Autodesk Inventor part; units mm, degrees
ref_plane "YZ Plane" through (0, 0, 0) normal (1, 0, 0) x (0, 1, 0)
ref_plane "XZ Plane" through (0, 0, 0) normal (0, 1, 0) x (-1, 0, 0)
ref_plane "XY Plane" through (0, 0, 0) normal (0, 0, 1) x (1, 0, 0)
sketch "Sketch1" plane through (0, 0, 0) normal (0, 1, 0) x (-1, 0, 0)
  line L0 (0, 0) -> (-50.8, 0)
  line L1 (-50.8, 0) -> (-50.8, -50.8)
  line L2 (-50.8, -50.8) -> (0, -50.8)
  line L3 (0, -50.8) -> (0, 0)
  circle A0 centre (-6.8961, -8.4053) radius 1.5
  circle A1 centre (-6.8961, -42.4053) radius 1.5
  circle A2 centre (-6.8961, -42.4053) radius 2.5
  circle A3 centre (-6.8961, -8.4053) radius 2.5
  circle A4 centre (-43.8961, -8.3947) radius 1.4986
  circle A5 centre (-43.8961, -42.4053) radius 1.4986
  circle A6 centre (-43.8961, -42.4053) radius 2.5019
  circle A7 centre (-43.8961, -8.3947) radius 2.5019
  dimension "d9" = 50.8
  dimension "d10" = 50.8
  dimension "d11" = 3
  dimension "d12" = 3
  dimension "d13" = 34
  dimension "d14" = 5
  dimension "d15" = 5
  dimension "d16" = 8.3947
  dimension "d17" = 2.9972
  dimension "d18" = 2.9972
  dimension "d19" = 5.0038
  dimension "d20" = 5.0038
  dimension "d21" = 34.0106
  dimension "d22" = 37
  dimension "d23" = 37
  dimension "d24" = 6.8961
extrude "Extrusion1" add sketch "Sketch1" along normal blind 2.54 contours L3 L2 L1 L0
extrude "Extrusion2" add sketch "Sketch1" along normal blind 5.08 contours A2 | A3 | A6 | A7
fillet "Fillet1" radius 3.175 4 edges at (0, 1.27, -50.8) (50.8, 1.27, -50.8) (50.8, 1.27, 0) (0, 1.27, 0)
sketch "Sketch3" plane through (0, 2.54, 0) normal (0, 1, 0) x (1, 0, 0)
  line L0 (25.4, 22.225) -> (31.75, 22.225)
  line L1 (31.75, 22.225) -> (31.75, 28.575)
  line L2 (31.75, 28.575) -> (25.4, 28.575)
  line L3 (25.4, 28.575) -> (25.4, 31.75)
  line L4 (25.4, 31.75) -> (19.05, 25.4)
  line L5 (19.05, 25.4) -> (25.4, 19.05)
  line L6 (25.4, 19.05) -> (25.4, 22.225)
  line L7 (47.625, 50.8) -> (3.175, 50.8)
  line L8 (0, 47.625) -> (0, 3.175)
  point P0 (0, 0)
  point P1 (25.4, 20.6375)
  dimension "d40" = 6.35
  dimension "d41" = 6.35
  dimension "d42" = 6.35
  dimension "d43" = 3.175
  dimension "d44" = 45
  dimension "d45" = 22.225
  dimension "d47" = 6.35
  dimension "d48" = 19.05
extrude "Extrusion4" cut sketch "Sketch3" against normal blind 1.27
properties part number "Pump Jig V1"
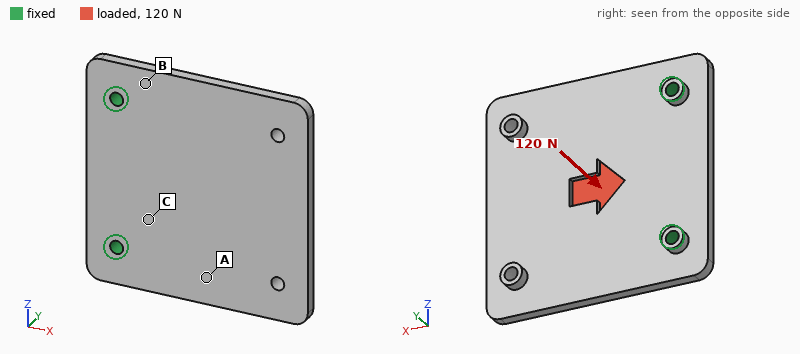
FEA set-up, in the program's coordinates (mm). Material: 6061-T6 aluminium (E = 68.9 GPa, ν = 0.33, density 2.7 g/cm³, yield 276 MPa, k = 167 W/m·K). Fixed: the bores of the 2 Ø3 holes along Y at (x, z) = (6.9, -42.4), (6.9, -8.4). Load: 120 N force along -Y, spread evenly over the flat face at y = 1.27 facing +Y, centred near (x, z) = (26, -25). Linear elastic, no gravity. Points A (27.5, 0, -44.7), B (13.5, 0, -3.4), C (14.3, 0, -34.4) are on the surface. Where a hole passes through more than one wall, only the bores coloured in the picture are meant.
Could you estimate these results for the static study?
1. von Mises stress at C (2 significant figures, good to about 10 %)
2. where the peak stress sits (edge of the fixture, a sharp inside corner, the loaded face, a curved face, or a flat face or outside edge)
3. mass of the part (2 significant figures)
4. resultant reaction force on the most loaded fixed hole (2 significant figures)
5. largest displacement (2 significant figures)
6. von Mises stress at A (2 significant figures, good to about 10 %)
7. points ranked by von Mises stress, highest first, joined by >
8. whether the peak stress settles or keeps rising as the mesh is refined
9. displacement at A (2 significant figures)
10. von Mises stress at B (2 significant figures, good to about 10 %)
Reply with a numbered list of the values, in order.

1. 22 MPa
2. edge of the fixture
3. 18 g
4. 62 N
5. 0.22 mm
6. 6.6 MPa
7. B > C > A
8. keeps rising
9. 0.071 mm
10. 33 MPa
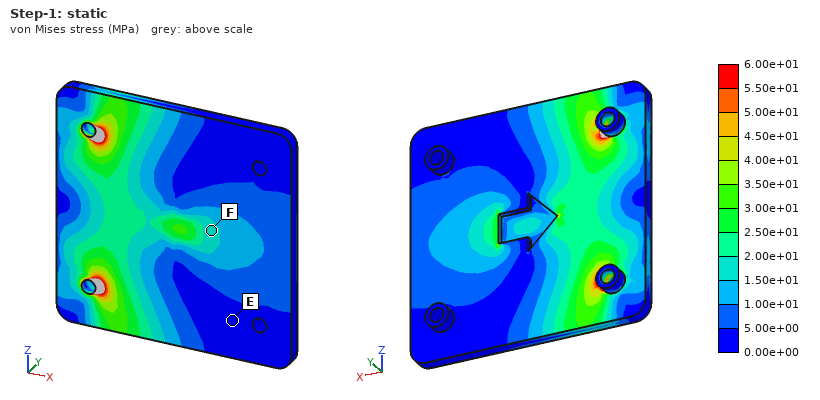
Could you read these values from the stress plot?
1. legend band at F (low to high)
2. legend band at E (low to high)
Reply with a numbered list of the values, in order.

1. 1.50e+01 to 2.00e+01 MPa
2. 0.00e+00 to 5.00e+00 MPa
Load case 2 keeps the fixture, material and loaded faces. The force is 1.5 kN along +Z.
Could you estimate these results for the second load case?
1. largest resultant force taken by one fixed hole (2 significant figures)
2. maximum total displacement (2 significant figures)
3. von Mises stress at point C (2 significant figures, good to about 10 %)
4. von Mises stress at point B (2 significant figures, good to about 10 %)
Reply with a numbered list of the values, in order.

1. 1.1 kN
2. 23 µm
3. 29 MPa
4. 13 MPa
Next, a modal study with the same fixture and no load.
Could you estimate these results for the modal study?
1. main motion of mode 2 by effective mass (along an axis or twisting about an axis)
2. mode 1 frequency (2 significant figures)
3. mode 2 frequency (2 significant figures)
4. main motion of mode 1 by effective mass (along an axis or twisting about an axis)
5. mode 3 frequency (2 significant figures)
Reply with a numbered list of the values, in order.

1. twisting about X
2. 1000 Hz
3. 2300 Hz
4. along Y
5. 6100 Hz
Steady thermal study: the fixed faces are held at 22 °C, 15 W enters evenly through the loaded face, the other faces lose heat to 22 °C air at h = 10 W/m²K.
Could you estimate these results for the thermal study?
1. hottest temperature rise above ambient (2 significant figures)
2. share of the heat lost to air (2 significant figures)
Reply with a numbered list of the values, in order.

1. 25 K
2. 4.6 %
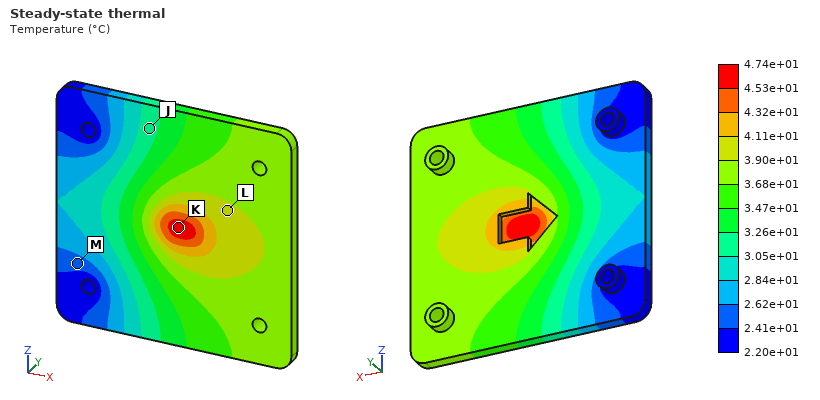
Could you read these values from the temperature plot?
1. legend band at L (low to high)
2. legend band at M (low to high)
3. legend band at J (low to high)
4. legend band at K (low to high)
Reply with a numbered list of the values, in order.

1. 3.90e+01 to 4.11e+01 °C
2. 2.41e+01 to 2.62e+01 °C
3. 3.05e+01 to 3.26e+01 °C
4. 4.53e+01 to 4.74e+01 °C
